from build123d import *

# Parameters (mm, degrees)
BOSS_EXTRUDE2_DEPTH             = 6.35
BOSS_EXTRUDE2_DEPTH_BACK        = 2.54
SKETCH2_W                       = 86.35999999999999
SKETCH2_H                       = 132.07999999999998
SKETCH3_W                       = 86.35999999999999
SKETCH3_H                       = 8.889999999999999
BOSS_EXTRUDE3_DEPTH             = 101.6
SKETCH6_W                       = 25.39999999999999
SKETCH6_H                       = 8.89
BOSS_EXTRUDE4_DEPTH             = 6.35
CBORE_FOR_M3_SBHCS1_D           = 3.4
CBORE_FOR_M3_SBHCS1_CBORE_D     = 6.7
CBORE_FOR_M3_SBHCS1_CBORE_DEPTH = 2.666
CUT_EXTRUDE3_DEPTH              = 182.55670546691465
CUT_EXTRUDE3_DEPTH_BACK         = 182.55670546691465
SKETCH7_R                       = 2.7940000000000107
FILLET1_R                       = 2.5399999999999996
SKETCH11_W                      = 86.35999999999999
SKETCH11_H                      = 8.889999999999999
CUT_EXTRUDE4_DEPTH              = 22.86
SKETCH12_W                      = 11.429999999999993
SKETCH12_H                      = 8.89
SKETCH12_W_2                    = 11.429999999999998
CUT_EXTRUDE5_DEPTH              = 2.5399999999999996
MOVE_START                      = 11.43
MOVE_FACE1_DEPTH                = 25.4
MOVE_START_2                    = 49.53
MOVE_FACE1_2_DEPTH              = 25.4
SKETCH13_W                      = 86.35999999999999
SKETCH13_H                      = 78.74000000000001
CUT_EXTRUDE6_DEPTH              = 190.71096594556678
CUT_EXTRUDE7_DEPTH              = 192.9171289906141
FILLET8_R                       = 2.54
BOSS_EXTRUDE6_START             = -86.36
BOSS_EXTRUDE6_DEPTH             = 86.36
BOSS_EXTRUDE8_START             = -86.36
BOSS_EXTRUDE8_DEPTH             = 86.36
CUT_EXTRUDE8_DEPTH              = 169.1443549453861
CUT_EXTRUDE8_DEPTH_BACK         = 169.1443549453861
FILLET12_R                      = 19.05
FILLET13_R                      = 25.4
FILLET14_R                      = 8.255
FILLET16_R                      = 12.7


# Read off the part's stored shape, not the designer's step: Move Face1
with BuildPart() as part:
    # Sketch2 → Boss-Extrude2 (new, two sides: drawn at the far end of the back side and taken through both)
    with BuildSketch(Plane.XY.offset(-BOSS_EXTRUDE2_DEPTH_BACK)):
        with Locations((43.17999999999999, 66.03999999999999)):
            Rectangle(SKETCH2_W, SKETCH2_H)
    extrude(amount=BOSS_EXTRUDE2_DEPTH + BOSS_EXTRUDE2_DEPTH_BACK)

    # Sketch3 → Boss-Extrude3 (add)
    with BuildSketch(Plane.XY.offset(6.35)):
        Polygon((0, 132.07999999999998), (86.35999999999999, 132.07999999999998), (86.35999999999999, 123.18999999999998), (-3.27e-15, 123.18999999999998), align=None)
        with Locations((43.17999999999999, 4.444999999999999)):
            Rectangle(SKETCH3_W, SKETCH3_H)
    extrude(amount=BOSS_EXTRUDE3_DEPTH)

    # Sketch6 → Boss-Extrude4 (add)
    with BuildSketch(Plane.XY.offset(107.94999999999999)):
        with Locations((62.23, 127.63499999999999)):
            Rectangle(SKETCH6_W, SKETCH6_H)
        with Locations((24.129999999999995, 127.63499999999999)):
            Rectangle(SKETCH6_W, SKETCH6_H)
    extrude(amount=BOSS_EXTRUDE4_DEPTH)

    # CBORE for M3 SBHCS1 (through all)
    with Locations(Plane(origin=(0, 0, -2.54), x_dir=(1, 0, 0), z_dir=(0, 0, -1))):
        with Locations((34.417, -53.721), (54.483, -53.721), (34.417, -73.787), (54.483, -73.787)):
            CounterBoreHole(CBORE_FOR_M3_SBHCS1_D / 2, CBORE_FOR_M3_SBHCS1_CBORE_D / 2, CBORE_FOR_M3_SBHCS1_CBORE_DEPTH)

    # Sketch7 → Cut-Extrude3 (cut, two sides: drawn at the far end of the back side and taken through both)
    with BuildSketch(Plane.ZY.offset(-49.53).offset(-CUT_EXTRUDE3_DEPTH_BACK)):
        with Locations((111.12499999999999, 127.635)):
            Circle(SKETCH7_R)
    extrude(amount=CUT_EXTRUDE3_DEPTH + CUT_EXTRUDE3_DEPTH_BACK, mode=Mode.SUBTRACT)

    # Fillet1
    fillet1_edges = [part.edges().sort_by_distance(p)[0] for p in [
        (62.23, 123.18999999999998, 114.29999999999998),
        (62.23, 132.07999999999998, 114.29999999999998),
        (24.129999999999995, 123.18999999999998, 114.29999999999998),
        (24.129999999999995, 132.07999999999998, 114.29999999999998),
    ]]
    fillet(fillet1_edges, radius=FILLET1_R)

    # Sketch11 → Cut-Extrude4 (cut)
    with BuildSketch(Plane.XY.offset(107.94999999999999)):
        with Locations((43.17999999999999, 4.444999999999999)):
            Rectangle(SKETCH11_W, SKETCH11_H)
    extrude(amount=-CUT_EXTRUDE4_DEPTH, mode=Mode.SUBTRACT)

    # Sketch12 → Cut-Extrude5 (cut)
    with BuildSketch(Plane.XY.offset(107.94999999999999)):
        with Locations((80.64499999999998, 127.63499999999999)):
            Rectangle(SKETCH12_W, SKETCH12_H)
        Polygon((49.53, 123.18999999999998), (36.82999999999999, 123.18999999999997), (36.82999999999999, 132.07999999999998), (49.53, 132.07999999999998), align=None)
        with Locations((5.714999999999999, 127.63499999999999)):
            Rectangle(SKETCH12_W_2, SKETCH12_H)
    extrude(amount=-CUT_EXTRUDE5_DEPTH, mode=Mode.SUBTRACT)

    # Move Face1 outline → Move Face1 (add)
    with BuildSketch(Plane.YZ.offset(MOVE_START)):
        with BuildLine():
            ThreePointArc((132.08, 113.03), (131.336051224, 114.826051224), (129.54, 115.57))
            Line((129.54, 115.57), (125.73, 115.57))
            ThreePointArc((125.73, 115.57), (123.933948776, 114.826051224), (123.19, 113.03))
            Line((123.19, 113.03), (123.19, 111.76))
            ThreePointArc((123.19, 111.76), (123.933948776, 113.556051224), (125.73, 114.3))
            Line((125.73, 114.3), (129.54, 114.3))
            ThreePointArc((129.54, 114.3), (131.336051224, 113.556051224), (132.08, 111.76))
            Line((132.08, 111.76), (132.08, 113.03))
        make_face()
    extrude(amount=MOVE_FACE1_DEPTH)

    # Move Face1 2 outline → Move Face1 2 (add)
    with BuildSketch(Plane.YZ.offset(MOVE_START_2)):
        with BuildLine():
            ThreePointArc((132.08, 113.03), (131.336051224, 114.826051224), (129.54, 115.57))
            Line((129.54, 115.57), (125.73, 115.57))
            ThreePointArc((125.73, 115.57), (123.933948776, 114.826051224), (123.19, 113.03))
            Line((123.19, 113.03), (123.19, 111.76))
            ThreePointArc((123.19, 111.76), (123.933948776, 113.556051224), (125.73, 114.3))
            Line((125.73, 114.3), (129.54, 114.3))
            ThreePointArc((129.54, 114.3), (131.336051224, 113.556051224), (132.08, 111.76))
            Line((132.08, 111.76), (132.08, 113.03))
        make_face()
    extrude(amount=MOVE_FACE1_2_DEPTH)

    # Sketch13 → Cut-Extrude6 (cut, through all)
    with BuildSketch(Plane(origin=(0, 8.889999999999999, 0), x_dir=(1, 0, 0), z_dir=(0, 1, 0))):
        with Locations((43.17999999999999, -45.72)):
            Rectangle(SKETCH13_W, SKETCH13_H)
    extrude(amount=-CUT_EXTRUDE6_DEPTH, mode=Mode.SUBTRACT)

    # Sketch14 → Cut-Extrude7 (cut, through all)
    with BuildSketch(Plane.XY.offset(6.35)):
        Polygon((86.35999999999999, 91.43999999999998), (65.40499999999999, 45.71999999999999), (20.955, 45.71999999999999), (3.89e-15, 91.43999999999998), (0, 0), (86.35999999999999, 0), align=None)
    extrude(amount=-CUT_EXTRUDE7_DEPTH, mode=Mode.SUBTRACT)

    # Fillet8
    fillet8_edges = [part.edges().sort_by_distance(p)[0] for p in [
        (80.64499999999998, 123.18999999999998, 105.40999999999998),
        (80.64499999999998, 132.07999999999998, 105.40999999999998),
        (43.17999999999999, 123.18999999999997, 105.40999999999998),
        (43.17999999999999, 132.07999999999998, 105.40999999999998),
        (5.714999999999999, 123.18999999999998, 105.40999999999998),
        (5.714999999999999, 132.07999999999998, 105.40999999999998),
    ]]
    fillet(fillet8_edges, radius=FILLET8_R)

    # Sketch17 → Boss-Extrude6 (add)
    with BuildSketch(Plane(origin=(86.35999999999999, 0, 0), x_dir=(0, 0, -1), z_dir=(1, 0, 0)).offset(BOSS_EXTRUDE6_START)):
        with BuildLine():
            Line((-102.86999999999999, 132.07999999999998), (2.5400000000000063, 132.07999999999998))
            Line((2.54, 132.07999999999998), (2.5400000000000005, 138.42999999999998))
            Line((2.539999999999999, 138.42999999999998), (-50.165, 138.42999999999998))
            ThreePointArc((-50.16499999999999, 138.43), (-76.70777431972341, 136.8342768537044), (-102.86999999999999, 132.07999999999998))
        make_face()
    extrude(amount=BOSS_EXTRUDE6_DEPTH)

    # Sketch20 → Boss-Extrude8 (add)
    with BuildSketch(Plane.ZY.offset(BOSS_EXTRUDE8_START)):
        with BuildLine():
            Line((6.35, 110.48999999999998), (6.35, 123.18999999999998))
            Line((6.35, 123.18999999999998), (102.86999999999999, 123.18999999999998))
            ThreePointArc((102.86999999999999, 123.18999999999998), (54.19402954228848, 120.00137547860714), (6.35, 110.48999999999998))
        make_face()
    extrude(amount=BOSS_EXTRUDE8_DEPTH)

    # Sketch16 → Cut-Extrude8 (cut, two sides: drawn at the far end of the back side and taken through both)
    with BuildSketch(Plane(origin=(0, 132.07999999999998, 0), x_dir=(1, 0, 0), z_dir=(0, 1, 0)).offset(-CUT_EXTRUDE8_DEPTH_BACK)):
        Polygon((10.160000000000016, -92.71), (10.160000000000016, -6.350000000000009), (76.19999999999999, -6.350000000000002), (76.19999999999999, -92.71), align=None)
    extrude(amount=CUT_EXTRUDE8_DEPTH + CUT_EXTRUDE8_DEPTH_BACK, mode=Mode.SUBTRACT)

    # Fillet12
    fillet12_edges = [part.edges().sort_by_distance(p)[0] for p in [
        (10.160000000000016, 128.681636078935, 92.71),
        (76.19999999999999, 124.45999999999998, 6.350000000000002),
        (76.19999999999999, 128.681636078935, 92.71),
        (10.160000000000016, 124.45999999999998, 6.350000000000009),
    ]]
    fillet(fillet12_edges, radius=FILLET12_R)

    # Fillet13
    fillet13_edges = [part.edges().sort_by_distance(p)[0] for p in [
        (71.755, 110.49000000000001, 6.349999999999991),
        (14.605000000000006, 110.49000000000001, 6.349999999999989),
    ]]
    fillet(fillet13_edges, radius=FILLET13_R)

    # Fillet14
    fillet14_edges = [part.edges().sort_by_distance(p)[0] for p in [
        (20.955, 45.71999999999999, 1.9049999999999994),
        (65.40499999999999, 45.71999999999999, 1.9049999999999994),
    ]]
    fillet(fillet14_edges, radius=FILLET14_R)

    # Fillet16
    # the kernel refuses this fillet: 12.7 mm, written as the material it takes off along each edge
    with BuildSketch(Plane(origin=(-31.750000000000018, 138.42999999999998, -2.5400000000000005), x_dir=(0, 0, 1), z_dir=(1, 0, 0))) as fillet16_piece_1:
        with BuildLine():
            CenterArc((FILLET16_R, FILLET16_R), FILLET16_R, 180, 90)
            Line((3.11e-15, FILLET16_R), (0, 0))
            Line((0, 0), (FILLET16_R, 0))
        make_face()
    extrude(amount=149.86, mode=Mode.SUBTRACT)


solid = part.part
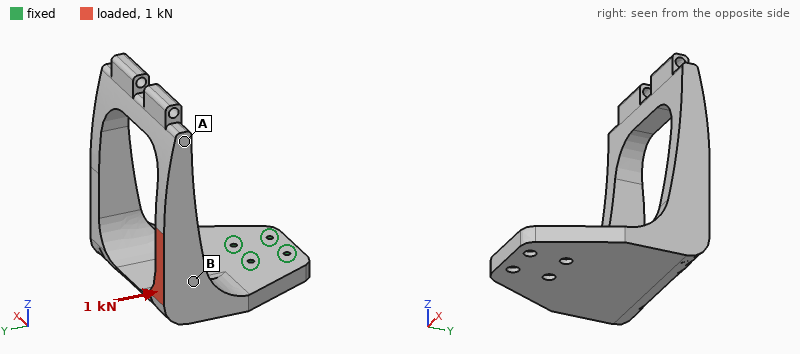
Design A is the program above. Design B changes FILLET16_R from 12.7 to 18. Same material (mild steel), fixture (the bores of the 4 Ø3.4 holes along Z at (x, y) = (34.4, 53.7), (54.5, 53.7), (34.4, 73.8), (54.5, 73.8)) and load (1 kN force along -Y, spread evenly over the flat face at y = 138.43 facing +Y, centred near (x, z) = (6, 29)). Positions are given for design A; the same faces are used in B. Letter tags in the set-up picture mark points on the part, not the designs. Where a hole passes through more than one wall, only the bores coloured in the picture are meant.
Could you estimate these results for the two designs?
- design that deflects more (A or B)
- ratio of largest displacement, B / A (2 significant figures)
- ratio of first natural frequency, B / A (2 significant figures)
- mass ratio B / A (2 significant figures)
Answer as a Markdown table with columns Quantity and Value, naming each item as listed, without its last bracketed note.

| Quantity | Value |
|---|---|
| design that deflects more | B |
| ratio of largest displacement, B / A | 1.1 |
| ratio of first natural frequency, B / A | 1.0 |
| mass ratio B / A | 0.98 |
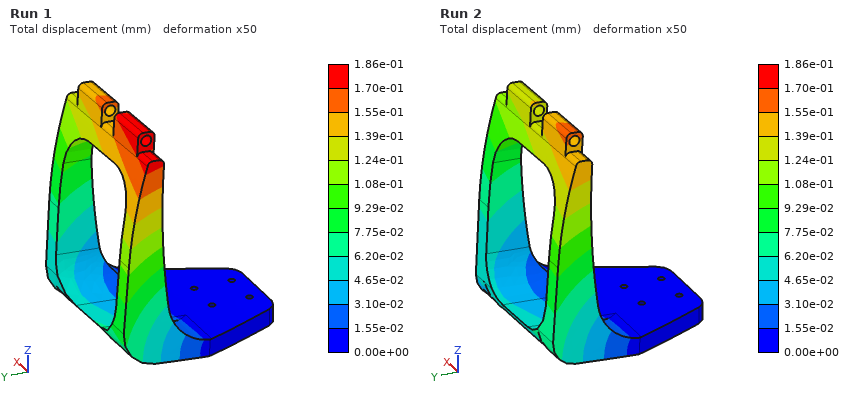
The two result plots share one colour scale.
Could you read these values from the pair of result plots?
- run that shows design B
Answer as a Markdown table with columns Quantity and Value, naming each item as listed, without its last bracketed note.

| Quantity | Value |
|---|---|
| run that shows design B | Run 1 |
